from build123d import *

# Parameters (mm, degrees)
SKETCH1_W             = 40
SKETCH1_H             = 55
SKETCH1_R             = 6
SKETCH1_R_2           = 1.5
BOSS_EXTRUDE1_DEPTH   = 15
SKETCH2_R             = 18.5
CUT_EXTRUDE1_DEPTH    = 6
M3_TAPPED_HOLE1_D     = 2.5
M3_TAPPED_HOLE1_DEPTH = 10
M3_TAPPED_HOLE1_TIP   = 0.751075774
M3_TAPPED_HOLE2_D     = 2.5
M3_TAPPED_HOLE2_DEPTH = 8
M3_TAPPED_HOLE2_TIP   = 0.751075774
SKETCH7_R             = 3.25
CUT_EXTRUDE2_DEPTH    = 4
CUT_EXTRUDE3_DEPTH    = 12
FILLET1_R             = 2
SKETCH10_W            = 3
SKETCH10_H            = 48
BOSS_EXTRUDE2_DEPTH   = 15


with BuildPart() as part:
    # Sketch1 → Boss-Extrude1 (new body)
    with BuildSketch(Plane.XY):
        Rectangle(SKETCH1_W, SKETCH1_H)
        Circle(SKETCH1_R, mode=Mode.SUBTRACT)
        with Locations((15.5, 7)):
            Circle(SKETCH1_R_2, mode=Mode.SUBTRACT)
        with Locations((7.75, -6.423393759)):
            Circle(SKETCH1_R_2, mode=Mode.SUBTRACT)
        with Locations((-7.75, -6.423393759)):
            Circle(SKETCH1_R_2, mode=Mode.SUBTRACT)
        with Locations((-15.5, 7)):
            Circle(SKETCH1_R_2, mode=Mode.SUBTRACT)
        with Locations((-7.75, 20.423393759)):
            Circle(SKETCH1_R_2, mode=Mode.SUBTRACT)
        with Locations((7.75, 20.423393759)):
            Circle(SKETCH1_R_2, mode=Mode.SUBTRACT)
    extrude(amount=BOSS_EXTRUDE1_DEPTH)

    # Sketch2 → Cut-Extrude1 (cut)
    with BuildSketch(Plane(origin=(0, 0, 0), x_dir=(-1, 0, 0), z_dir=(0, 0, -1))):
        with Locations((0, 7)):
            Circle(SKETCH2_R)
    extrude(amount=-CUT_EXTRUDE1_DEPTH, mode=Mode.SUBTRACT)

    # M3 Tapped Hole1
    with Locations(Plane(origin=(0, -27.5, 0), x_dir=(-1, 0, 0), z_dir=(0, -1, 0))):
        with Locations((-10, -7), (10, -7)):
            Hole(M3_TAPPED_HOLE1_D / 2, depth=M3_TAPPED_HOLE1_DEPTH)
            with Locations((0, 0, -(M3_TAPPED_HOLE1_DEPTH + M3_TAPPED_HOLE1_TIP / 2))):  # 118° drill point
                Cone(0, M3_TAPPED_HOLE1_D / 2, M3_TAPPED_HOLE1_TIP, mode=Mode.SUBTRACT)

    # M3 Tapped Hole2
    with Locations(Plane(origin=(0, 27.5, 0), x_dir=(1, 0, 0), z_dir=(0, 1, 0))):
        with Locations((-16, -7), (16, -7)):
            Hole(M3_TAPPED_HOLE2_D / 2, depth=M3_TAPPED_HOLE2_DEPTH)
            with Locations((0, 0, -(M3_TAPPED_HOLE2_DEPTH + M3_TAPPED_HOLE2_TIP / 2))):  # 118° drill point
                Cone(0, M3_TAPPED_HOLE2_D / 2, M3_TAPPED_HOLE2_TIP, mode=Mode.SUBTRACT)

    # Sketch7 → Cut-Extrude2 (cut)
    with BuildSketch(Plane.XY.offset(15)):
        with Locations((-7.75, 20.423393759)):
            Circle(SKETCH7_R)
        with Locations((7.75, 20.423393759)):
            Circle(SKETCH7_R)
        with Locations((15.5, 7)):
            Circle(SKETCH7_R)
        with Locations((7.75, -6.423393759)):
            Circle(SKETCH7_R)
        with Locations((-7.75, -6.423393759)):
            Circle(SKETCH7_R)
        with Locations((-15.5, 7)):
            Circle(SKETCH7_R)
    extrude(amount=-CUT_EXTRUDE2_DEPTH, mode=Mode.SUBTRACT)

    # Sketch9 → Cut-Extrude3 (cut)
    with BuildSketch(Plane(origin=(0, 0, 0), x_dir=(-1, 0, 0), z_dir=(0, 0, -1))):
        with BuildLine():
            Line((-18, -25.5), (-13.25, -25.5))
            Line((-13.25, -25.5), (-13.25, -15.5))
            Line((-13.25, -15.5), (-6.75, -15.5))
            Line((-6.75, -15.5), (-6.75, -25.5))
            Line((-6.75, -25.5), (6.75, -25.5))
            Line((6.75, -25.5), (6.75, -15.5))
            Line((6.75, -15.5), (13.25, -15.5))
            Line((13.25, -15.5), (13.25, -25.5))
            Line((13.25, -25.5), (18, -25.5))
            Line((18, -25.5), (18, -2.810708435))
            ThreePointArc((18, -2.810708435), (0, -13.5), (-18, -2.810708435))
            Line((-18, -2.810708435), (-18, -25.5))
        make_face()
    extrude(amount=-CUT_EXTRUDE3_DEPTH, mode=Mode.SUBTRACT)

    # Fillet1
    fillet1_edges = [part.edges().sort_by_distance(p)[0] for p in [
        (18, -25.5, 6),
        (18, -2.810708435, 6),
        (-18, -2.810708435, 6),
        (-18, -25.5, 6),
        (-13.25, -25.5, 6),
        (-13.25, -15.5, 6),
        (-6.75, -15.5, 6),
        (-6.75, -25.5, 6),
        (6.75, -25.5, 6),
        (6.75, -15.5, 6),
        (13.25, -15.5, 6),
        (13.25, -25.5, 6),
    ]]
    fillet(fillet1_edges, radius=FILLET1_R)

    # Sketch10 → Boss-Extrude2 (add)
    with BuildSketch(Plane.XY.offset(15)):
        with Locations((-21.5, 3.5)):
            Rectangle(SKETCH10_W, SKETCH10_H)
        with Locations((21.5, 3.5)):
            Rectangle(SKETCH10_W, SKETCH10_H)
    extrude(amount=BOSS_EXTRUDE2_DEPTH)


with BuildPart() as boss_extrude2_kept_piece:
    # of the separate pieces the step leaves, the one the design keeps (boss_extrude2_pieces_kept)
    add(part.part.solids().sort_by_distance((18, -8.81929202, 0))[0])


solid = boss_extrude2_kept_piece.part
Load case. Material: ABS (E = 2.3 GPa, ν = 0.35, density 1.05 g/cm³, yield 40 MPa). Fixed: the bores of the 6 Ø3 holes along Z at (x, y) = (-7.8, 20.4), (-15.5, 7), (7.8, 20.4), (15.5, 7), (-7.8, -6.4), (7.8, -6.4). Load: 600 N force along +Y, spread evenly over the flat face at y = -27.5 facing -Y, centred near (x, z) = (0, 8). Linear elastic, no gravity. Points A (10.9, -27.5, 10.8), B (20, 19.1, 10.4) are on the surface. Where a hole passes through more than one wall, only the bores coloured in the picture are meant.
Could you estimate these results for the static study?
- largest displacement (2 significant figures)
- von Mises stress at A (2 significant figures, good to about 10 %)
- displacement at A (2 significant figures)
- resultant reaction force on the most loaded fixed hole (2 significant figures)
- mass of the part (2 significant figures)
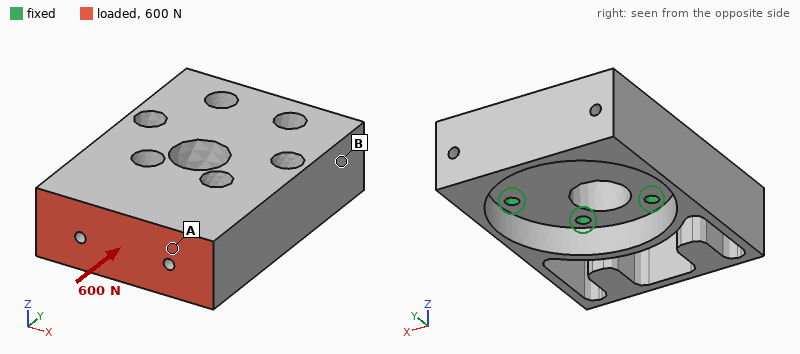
0.59 mm
6.3 MPa
0.29 mm
150 N
21 g
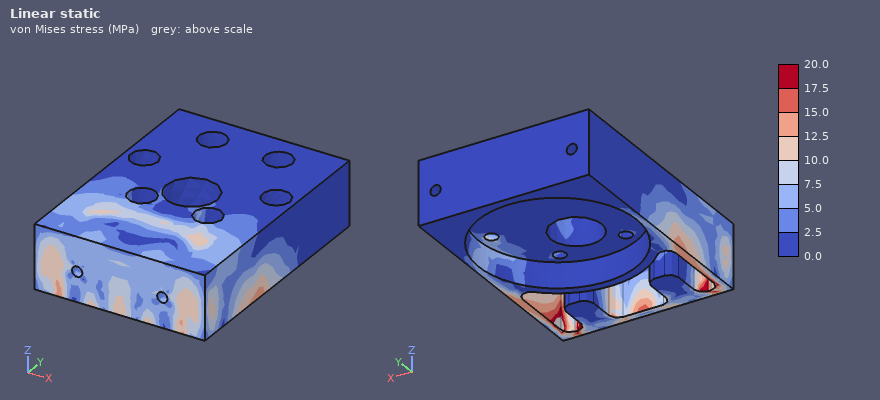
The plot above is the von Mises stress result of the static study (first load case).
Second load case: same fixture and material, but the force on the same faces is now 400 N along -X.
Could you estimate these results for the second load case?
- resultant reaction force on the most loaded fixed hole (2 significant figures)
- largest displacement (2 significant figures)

290 N
0.48 mm
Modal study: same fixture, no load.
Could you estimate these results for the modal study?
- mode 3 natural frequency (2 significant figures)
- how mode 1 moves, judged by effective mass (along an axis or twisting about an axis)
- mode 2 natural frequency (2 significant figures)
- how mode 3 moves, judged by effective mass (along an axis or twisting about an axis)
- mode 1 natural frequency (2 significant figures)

5000 Hz
along Z
2400 Hz
along X
2100 Hz
